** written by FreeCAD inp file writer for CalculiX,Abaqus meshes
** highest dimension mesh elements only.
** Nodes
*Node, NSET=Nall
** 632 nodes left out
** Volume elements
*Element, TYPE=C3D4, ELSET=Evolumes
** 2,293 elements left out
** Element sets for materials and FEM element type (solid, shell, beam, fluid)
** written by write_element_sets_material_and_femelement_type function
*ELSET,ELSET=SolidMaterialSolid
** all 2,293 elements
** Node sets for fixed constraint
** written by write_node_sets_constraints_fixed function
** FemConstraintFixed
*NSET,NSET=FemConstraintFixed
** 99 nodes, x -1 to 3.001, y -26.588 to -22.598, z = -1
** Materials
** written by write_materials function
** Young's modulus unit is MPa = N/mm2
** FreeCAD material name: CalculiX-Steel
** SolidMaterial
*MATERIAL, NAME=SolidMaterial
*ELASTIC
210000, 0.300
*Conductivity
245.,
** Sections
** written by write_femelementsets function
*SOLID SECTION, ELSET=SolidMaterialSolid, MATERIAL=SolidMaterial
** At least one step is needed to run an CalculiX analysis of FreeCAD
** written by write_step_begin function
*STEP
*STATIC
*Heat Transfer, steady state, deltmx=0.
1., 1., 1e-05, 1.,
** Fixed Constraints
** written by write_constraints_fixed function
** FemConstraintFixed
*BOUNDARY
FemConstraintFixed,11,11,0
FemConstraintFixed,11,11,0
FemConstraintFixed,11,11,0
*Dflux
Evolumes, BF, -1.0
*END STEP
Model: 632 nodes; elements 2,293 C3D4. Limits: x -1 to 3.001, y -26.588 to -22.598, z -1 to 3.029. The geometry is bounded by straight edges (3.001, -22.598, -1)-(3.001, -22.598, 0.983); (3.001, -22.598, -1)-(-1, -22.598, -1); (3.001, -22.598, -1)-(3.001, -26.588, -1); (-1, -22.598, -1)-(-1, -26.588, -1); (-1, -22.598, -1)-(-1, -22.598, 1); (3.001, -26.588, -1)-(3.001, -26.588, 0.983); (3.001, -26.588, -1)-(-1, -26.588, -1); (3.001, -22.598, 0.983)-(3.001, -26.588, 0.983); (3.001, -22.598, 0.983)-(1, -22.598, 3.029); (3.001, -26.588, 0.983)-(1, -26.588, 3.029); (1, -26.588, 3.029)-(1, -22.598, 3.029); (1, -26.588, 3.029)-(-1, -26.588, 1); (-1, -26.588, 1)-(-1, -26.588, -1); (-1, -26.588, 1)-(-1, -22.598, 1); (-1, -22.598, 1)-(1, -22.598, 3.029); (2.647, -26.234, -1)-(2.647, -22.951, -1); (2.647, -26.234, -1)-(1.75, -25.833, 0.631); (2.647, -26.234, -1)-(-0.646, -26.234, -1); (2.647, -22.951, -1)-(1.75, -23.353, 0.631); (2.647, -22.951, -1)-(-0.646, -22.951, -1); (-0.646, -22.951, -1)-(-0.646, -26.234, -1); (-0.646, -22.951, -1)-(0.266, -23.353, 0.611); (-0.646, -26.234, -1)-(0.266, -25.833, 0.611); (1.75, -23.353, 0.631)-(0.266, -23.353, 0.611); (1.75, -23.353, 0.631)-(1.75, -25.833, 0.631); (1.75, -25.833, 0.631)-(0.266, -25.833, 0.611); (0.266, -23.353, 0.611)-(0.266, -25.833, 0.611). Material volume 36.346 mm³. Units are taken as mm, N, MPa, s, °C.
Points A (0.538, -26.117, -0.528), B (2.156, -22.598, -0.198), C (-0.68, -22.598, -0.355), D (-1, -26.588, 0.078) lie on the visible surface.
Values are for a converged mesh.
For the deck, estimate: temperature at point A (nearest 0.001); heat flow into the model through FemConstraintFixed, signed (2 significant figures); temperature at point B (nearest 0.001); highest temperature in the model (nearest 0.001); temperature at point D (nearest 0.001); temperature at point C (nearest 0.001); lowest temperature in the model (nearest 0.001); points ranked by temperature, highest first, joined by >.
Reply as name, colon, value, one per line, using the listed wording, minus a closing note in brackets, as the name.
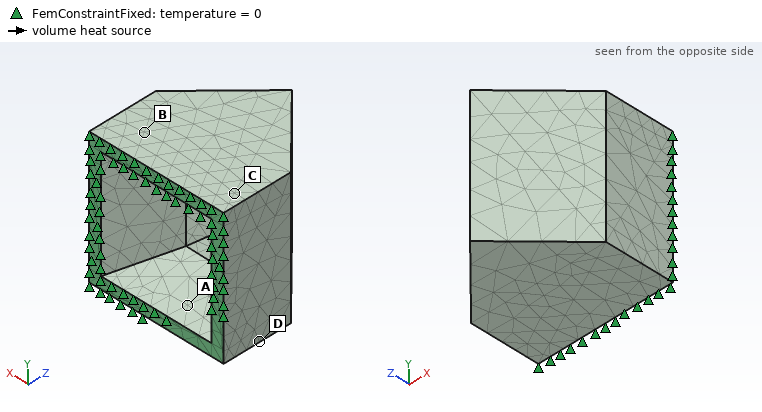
temperature at point A: -0.012 °C
heat flow into the model through FemConstraintFixed, signed: 36 mW
temperature at point B: -0.016 °C
highest temperature in the model: 0.000 °C
temperature at point D: -0.019 °C
temperature at point C: -0.013 °C
lowest temperature in the model: -0.034 °C
points ranked by temperature, highest first, joined by >: A > C > B > D
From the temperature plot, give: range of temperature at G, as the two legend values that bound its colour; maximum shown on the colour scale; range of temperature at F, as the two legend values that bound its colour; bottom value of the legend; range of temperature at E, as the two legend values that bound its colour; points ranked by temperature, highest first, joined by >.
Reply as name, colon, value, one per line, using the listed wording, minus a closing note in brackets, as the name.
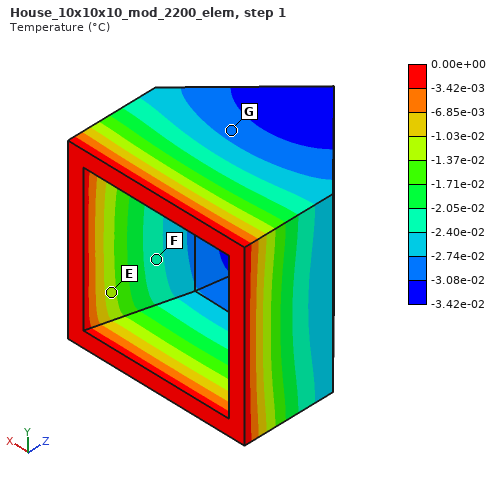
range of temperature at G, as the two legend values that bound its colour: -3.08e-02 to -2.74e-02 °C
maximum shown on the colour scale: 0.00e+00 °C
range of temperature at F, as the two legend values that bound its colour: -2.40e-02 to -2.05e-02 °C
bottom value of the legend: -3.42e-02 °C
range of temperature at E, as the two legend values that bound its colour: -1.37e-02 to -1.03e-02 °C
points ranked by temperature, highest first, joined by >: E > F > G
